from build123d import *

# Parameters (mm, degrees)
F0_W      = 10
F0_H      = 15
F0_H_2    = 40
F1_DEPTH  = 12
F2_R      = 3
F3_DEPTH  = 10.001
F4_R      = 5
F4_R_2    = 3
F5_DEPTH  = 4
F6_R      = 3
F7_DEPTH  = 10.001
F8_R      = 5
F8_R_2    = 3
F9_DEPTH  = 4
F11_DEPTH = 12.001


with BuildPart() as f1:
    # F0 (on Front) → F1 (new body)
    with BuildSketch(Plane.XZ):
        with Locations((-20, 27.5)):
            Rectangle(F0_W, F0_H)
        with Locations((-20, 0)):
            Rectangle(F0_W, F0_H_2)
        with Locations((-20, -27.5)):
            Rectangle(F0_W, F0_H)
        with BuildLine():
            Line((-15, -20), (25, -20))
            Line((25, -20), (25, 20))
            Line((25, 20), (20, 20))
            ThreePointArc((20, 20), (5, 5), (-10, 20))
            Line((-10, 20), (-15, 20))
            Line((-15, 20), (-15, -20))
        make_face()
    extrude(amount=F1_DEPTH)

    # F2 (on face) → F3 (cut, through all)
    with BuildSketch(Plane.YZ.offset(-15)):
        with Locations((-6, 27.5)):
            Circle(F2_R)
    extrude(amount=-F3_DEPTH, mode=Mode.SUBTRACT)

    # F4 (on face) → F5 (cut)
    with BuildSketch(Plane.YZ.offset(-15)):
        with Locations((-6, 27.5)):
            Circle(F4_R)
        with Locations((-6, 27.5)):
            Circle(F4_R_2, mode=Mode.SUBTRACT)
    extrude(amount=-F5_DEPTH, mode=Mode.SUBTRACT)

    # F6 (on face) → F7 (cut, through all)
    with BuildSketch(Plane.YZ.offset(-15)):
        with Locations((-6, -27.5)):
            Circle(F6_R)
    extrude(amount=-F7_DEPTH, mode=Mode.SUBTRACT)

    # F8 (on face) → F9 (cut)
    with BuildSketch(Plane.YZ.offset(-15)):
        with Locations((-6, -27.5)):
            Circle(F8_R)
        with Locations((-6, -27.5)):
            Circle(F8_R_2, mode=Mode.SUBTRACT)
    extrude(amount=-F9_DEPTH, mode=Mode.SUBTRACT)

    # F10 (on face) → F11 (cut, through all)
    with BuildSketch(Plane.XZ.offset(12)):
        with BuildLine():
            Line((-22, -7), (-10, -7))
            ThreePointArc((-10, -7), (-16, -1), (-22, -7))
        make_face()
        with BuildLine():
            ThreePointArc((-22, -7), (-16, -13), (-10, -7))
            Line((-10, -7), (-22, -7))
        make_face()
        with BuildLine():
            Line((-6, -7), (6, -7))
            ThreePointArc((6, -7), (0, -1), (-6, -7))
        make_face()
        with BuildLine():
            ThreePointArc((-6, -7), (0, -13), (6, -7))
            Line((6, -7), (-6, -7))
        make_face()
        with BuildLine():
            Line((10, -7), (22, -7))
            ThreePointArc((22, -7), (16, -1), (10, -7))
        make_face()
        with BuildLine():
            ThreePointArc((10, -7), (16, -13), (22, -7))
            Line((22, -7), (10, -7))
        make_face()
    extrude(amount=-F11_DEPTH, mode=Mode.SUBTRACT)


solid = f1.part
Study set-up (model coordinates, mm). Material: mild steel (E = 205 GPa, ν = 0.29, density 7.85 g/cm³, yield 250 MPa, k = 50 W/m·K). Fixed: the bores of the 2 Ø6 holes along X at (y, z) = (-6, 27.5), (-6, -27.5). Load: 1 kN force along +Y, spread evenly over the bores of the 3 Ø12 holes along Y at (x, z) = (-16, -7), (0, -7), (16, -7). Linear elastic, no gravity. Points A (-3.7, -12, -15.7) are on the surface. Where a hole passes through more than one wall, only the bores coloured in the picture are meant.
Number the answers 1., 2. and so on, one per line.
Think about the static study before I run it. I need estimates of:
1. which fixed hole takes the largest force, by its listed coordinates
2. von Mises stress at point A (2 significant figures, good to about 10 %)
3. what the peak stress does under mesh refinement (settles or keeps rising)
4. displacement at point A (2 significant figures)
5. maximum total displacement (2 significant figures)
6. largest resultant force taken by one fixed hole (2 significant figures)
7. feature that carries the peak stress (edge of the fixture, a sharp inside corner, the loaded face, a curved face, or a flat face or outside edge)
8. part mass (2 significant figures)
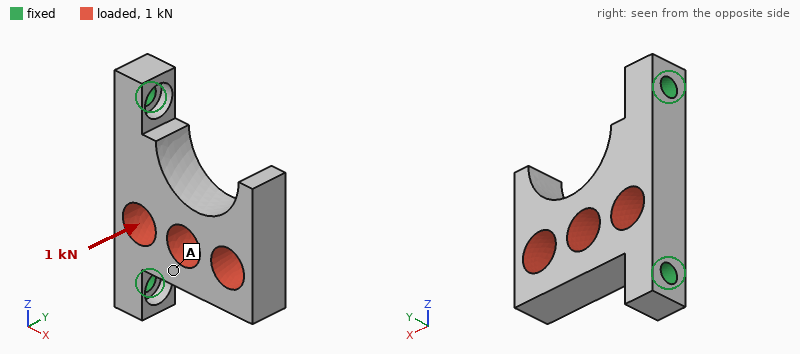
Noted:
1. (-6, -27.5)
2. 18 MPa
3. keeps rising
4. 23 µm
5. 63 µm
6. 660 N
7. edge of the fixture
8. 140 g
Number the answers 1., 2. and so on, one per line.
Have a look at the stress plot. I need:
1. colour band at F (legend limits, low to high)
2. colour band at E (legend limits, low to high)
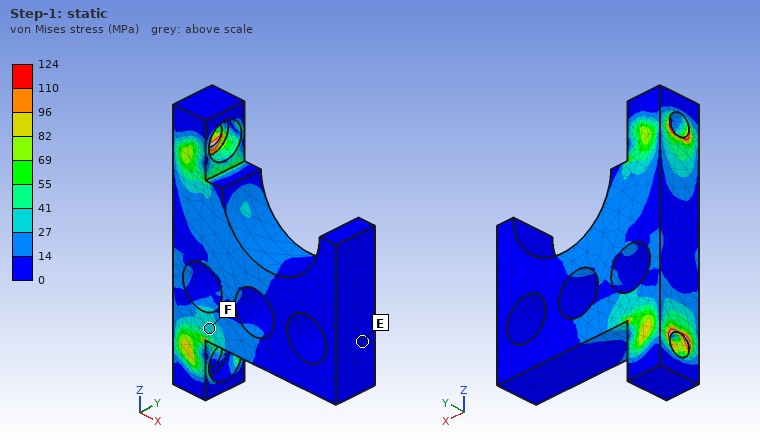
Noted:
1. 27 to 41 MPa
2. 0 to 14 MPa
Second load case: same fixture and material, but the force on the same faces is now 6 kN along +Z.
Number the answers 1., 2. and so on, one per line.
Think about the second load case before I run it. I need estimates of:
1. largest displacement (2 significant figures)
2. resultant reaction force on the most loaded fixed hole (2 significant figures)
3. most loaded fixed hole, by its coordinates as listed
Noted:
1. 37 µm
2. 4.5 kN
3. (-6, 27.5)
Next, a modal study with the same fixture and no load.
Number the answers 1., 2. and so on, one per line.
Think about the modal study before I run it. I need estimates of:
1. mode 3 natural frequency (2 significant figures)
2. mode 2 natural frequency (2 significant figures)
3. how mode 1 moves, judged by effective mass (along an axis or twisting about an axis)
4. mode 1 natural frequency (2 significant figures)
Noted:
1. 6800 Hz
2. 6700 Hz
3. along Y
4. 2200 Hz
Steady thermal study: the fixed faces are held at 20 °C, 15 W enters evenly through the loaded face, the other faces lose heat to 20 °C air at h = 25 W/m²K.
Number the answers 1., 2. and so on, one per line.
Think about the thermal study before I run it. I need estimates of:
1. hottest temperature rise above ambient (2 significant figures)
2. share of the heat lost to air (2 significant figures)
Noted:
1. 34 K
2. 19 %
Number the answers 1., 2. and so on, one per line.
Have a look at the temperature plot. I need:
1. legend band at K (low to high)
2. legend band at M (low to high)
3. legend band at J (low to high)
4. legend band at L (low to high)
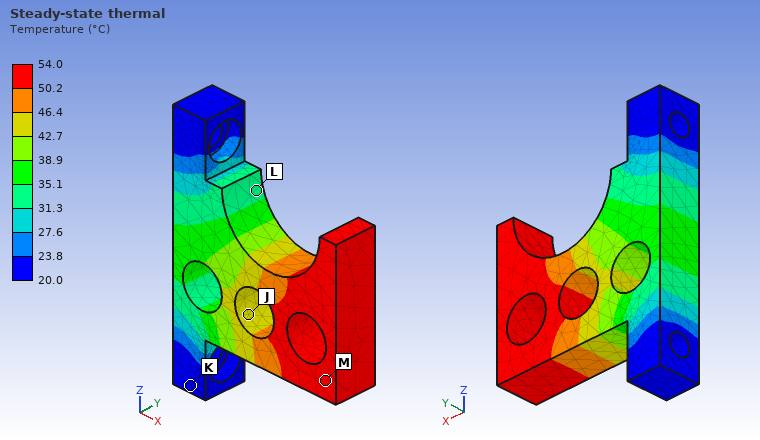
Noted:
1. 20.0 to 23.8 °C
2. 50.2 to 54.0 °C
3. 42.7 to 46.4 °C
4. 31.3 to 35.1 °C
